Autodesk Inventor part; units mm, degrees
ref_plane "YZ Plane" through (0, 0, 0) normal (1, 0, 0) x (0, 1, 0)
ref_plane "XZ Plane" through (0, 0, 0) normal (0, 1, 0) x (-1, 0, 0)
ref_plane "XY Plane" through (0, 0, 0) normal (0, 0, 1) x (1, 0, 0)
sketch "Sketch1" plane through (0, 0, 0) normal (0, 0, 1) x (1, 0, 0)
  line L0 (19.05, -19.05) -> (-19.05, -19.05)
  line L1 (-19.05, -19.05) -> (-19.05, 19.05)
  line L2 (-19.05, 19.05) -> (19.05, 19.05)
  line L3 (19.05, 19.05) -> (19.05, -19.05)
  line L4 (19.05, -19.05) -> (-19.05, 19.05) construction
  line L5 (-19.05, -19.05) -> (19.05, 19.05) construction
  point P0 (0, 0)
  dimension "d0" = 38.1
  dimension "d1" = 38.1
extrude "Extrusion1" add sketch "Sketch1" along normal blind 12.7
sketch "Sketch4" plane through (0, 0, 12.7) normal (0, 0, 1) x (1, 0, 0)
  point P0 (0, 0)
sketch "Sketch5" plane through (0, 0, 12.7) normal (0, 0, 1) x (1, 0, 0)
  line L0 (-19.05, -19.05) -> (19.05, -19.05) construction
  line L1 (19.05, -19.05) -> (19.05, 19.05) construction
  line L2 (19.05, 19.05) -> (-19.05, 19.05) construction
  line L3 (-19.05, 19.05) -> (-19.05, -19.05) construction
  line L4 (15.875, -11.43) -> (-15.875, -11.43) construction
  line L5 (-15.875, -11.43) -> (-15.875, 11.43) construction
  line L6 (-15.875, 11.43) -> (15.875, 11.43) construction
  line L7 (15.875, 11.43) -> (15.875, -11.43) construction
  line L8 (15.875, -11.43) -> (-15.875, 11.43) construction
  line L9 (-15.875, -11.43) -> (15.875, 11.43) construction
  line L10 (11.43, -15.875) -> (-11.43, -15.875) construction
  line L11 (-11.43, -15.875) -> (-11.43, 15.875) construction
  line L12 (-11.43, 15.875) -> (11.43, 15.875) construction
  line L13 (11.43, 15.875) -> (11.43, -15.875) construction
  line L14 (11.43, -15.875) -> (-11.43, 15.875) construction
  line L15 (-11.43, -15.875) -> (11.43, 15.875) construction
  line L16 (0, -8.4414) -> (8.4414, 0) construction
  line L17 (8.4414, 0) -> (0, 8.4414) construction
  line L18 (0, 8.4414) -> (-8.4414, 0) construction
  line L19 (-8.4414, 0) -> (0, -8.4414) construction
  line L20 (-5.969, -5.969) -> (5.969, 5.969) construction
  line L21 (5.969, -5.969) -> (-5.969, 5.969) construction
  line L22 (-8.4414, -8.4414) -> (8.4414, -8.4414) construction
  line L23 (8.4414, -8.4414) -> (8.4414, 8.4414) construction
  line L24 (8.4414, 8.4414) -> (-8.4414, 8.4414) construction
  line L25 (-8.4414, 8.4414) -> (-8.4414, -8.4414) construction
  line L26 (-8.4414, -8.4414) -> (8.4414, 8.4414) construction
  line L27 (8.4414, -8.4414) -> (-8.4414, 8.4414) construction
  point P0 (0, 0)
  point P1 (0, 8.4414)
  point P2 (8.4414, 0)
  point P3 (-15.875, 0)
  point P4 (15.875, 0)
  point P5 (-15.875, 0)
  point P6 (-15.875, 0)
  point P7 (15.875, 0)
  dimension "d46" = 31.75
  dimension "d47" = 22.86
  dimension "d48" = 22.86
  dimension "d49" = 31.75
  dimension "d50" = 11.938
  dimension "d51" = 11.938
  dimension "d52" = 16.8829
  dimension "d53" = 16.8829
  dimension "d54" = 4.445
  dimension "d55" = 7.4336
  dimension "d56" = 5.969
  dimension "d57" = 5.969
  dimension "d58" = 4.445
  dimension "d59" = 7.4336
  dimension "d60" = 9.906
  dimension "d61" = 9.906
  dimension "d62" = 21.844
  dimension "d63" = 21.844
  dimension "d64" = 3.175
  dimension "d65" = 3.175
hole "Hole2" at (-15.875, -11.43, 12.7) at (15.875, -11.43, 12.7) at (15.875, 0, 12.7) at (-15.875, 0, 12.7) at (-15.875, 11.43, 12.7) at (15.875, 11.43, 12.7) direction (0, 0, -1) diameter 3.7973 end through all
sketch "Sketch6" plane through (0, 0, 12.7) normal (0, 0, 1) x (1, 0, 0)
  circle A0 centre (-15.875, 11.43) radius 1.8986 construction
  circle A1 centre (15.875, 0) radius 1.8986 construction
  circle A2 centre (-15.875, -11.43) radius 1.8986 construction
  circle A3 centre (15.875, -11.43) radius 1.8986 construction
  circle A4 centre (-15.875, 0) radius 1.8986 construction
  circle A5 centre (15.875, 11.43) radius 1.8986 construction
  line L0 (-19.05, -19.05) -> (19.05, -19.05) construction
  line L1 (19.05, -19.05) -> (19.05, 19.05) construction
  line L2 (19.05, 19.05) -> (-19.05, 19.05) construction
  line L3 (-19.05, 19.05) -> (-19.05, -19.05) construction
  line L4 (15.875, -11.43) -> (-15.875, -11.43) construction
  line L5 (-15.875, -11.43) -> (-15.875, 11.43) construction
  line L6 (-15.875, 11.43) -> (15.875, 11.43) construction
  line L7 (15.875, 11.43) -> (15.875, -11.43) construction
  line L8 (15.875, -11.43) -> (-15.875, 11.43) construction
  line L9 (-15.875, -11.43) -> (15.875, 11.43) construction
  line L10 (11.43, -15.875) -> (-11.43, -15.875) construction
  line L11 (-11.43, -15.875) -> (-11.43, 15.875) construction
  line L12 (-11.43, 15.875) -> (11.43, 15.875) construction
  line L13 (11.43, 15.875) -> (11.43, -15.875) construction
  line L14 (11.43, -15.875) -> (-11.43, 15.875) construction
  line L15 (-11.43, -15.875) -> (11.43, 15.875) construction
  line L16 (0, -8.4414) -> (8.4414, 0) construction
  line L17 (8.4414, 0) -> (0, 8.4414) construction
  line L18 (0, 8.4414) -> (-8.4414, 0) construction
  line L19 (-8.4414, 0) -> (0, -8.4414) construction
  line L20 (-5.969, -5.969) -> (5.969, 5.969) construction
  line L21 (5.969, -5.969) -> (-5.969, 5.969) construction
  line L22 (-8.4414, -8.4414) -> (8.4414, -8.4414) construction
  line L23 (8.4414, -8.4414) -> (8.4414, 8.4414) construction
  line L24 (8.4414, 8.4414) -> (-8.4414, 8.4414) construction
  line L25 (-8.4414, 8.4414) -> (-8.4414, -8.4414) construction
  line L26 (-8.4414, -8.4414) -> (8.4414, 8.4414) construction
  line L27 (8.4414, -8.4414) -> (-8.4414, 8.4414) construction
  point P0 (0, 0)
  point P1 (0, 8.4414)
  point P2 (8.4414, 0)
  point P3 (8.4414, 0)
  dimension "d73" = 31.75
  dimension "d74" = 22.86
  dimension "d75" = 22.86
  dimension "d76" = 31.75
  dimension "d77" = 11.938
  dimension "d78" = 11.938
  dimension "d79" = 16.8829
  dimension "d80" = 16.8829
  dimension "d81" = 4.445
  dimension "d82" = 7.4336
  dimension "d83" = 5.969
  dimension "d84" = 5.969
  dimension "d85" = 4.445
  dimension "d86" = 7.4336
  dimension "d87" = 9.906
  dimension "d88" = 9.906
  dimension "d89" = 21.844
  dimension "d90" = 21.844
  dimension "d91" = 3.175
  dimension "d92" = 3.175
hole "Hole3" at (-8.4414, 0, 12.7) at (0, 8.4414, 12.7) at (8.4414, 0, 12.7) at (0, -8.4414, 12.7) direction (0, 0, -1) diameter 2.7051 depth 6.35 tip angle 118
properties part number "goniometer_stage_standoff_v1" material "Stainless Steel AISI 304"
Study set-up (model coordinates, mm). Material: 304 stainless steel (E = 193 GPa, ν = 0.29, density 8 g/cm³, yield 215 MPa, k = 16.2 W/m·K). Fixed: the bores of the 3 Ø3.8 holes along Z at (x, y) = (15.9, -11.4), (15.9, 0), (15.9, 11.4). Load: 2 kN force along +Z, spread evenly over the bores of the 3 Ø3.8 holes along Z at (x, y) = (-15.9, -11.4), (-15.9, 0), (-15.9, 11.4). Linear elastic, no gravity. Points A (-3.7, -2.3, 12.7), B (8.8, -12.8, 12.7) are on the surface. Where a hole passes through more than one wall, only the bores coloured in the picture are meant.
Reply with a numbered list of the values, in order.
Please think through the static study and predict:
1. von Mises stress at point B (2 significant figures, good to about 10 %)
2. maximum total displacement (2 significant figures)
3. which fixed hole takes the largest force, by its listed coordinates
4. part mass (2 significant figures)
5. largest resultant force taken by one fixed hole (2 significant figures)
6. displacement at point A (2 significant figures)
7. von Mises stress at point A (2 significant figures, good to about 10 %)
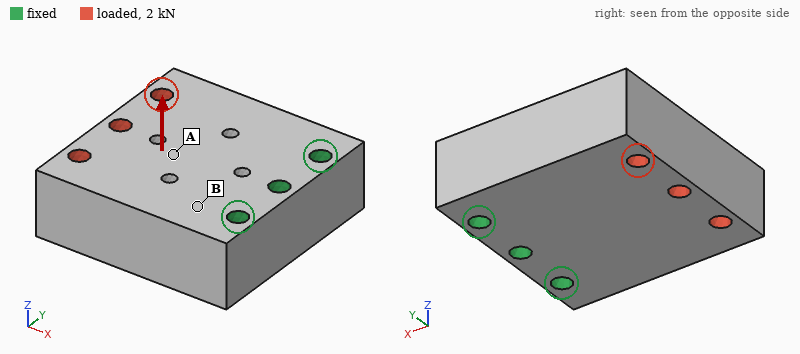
1. 51 MPa
2. 24 µm
3. (15.9, 0)
4. 140 g
5. 880 N
6. 11 µm
7. 24 MPa
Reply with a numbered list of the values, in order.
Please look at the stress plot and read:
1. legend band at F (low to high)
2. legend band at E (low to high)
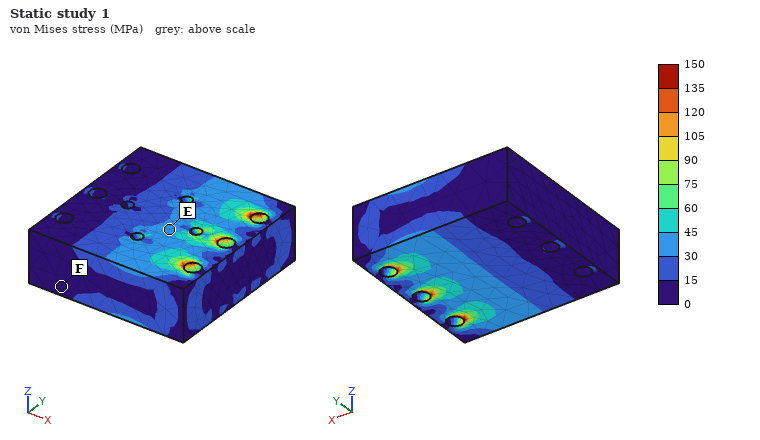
1. 0 to 15 MPa
2. 30 to 45 MPa
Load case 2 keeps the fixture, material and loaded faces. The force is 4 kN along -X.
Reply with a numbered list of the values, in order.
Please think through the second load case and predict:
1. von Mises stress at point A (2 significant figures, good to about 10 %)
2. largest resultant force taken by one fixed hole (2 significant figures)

1. 11 MPa
2. 1.4 kN
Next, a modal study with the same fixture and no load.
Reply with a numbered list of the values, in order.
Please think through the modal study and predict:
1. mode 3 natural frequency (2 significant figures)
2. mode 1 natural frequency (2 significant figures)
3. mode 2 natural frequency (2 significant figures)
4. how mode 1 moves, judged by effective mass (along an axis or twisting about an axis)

1. 14 kHz
2. 7700 Hz
3. 14 kHz
4. along Z
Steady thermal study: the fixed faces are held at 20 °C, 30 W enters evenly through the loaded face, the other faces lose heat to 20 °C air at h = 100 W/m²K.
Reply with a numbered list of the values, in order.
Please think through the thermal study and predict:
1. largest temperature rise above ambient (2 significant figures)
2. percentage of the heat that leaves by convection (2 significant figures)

1. 84 K
2. 54 %
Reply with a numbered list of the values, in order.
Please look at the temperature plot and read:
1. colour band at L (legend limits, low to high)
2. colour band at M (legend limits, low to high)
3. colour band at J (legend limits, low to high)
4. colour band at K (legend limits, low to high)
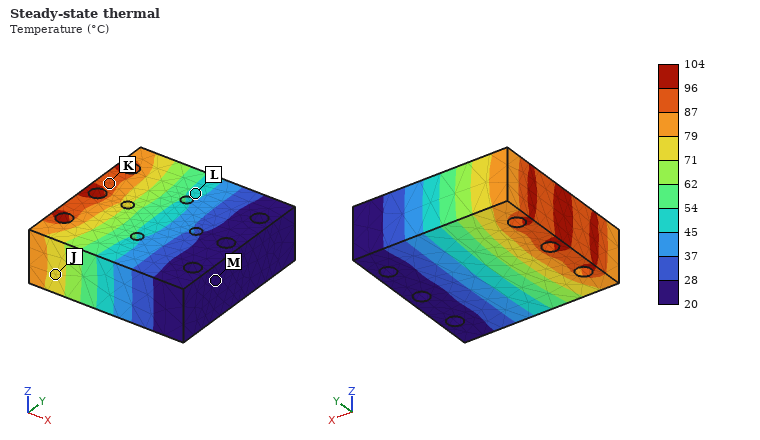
1. 45 to 54 °C
2. 20 to 28 °C
3. 71 to 79 °C
4. 87 to 96 °C
